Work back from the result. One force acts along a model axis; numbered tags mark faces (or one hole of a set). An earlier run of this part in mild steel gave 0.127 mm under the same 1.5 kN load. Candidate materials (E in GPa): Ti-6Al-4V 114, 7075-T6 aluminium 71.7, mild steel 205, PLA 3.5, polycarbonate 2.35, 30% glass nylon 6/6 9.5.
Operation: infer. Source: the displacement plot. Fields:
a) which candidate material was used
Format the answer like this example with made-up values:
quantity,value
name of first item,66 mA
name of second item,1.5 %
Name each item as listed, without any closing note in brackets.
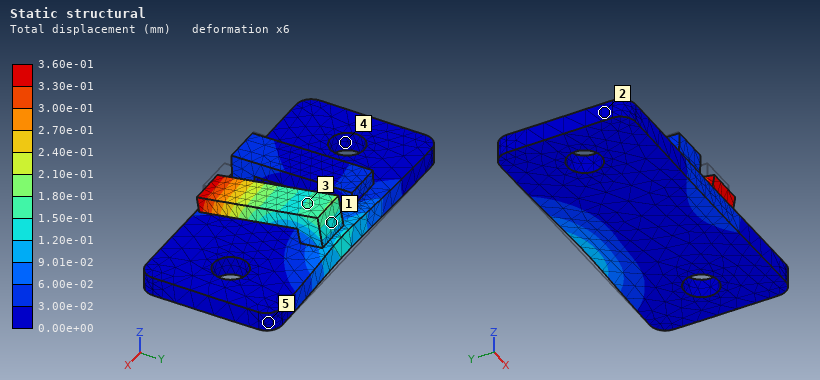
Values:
quantity,value
which candidate material was used,7075-T6 aluminium
